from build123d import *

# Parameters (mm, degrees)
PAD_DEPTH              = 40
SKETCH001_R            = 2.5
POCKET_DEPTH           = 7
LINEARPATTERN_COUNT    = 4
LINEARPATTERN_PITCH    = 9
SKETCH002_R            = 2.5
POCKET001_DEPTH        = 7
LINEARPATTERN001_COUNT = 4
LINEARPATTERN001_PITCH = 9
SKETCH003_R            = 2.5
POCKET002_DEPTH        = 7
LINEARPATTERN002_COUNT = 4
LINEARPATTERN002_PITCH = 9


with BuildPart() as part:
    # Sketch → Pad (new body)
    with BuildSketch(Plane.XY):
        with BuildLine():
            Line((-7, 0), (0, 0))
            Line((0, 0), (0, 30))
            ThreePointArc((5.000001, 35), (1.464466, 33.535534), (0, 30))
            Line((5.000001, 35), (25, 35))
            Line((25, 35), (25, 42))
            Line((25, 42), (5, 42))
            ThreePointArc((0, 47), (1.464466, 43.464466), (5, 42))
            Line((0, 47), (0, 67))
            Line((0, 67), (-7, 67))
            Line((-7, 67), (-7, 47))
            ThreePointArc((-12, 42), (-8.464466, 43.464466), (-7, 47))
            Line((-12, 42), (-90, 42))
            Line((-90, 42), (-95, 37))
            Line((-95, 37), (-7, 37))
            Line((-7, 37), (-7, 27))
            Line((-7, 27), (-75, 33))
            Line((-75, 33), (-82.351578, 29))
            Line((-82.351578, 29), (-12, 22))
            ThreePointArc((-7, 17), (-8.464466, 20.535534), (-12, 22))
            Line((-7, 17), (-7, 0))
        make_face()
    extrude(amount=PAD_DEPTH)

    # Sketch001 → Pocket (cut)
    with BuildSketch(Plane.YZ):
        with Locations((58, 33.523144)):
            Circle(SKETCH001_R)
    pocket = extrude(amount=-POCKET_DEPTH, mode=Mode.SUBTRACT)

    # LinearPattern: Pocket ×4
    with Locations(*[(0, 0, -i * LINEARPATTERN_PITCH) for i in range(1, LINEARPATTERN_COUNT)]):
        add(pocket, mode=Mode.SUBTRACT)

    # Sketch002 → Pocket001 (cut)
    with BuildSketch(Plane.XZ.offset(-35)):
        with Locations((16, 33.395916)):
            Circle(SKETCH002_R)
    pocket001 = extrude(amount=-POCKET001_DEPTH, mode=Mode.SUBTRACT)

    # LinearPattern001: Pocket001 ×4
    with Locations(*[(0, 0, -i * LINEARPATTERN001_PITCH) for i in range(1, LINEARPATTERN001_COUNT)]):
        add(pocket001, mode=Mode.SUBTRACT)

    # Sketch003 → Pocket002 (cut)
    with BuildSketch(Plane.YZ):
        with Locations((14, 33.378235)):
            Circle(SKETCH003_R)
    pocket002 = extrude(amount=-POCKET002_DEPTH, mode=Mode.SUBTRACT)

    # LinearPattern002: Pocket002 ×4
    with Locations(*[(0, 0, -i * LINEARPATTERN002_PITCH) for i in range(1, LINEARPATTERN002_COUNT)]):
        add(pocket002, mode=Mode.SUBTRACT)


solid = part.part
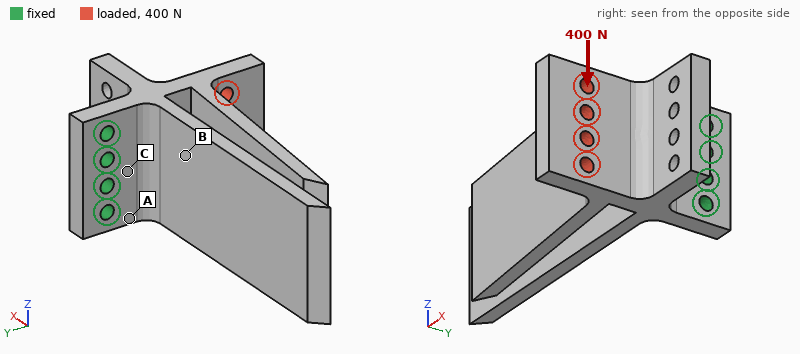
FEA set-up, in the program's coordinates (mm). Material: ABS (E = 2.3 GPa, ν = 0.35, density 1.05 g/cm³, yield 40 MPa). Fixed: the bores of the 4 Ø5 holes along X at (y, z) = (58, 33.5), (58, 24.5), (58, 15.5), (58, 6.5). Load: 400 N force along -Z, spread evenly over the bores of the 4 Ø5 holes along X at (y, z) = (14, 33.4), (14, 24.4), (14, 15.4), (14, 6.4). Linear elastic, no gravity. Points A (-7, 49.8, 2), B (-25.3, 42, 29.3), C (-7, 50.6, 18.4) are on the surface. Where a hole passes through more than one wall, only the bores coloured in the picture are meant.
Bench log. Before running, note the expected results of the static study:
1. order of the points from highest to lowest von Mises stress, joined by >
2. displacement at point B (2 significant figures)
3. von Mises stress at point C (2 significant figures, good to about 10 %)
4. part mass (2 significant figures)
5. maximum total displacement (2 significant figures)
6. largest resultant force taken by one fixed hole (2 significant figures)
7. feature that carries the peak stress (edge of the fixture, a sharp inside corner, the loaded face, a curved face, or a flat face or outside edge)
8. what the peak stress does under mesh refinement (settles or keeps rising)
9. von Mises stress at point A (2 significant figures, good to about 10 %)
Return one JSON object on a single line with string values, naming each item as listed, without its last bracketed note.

{"order of the points from highest to lowest von Mises stress, joined by >": "A > C > B", "displacement at point B": "0.060 mm", "von Mises stress at point C": "3.8 MPa", "part mass": "59 g", "maximum total displacement": "0.28 mm", "largest resultant force taken by one fixed hole": "560 N", "feature that carries the peak stress": "edge of the fixture", "what the peak stress does under mesh refinement": "keeps rising", "von Mises stress at point A": "6.0 MPa"}
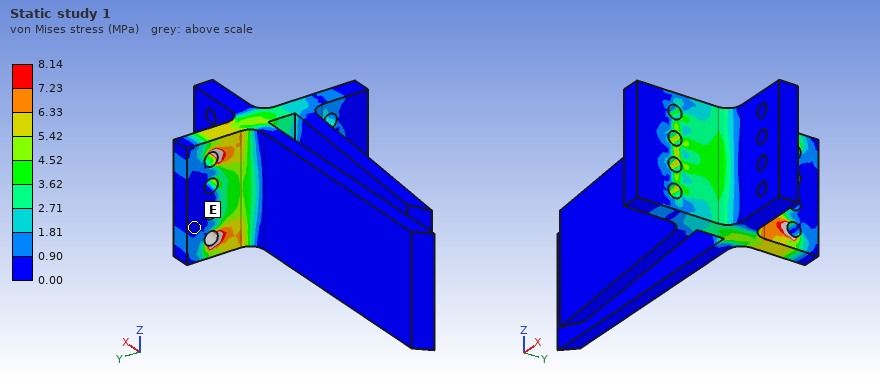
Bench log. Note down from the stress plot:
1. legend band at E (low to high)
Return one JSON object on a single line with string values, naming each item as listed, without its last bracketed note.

{"legend band at E": "0.00 to 0.90 MPa"}
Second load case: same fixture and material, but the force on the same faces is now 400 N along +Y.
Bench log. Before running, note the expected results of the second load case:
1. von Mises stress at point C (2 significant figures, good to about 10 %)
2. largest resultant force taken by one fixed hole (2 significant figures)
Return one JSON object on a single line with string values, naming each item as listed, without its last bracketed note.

{"von Mises stress at point C": "1.3 MPa", "largest resultant force taken by one fixed hole": "120 N"}
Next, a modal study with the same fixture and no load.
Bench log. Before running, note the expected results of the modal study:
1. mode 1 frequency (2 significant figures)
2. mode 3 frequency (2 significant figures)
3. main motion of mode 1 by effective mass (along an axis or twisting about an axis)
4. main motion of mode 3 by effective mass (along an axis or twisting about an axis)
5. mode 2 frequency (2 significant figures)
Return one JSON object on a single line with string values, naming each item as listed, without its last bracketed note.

{"mode 1 frequency": "150 Hz", "mode 3 frequency": "390 Hz", "main motion of mode 1 by effective mass": "along Y", "main motion of mode 3 by effective mass": "along Z", "mode 2 frequency": "210 Hz"}
